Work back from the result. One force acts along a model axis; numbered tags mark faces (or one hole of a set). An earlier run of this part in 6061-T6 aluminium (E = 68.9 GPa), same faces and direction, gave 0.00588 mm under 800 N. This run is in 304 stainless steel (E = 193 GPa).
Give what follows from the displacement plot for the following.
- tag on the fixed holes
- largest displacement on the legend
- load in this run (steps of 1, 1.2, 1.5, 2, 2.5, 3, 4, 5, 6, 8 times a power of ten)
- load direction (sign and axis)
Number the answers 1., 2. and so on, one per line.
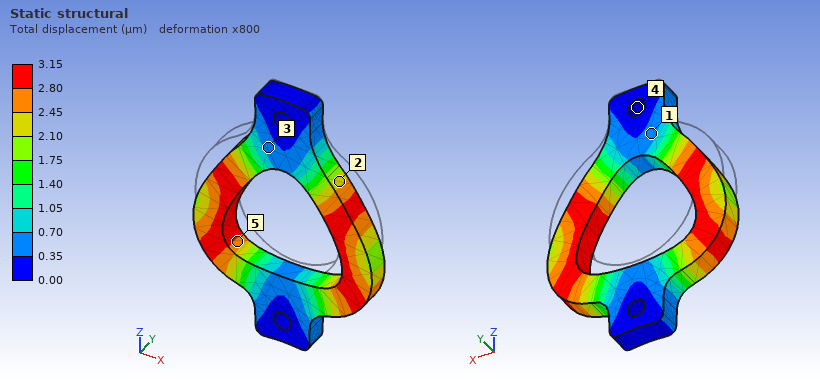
1. 4
2. 3.15 µm
3. 1.2 kN
4. -Z
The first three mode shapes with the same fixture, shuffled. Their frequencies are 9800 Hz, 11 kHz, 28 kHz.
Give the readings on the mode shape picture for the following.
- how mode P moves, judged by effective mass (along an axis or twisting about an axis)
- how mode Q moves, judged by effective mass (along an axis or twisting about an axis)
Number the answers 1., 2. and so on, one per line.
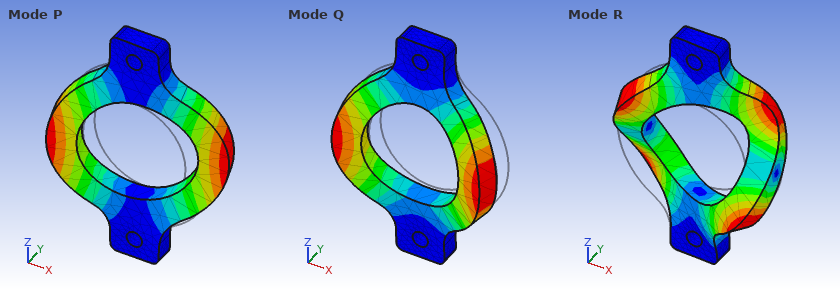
1. twisting about Z
2. along Y
